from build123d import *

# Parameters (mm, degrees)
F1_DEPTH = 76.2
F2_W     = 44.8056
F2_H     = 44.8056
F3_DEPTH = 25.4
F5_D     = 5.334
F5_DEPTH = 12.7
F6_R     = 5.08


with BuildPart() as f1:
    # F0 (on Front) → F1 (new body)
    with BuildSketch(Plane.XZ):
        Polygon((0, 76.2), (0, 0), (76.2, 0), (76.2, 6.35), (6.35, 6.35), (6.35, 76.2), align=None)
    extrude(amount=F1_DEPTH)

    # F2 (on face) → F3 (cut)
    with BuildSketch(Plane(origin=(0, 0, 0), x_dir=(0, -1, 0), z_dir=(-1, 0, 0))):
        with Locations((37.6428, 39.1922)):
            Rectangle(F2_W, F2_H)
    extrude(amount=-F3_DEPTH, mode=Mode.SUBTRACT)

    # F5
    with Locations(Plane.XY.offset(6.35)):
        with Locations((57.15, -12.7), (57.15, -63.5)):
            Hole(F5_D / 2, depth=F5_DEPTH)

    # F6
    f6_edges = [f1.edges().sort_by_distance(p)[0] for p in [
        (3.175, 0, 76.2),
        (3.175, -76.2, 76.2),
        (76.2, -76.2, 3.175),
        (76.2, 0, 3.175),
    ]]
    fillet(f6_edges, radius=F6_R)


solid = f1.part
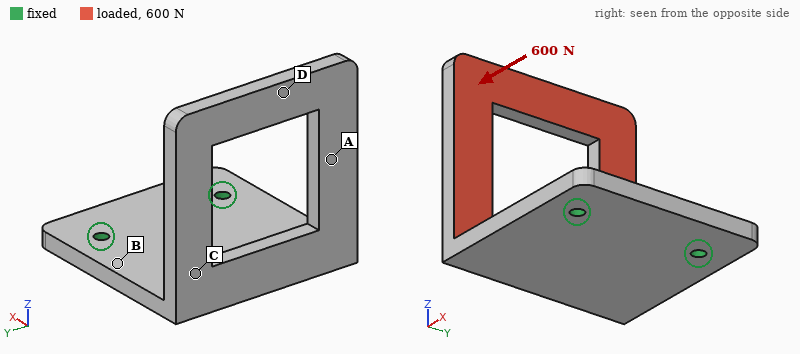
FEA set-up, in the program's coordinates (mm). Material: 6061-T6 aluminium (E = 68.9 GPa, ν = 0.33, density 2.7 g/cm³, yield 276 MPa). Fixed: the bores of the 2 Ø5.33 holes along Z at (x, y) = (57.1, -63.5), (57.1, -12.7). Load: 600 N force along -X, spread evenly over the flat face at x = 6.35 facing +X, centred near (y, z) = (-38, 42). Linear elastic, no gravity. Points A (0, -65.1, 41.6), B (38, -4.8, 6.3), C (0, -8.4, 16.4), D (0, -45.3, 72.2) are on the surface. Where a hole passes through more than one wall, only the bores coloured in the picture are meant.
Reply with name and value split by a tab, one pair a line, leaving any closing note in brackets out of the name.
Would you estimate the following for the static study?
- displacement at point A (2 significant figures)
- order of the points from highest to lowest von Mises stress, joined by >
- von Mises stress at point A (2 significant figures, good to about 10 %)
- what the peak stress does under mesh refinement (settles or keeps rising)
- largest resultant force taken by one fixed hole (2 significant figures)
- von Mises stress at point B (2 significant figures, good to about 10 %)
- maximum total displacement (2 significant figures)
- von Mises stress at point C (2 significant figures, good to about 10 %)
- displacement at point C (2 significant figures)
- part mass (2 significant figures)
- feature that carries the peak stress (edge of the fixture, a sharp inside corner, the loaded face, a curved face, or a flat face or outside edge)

displacement at point A	0.76 mm
order of the points from highest to lowest von Mises stress, joined by >	C > B > A > D
von Mises stress at point A	32 MPa
what the peak stress does under mesh refinement	keeps rising
largest resultant force taken by one fixed hole	310 N
von Mises stress at point B	50 MPa
maximum total displacement	1.5 mm
von Mises stress at point C	69 MPa
displacement at point C	0.41 mm
part mass	160 g
feature that carries the peak stress	edge of the fixture
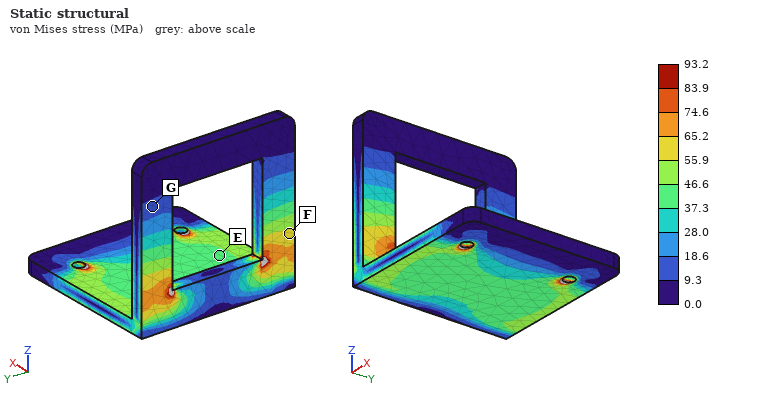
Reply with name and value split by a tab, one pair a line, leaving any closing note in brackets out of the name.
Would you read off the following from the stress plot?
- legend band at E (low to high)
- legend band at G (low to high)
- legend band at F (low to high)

legend band at E	37.3 to 46.6 MPa
legend band at G	9.3 to 18.6 MPa
legend band at F	55.9 to 65.2 MPa
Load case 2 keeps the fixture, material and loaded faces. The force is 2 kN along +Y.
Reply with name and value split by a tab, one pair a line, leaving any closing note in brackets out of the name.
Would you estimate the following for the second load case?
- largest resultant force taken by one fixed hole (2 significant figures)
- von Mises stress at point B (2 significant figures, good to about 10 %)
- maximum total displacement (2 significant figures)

largest resultant force taken by one fixed hole	2.6 kN
von Mises stress at point B	87 MPa
maximum total displacement	1.4 mm
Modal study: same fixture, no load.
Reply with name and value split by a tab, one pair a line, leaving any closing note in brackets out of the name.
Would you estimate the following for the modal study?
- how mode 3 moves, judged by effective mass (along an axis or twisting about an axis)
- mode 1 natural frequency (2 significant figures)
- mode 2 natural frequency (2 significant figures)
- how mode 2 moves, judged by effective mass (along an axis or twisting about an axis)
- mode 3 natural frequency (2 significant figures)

how mode 3 moves, judged by effective mass	along Z
mode 1 natural frequency	460 Hz
mode 2 natural frequency	860 Hz
how mode 2 moves, judged by effective mass	along Y
mode 3 natural frequency	1100 Hz
